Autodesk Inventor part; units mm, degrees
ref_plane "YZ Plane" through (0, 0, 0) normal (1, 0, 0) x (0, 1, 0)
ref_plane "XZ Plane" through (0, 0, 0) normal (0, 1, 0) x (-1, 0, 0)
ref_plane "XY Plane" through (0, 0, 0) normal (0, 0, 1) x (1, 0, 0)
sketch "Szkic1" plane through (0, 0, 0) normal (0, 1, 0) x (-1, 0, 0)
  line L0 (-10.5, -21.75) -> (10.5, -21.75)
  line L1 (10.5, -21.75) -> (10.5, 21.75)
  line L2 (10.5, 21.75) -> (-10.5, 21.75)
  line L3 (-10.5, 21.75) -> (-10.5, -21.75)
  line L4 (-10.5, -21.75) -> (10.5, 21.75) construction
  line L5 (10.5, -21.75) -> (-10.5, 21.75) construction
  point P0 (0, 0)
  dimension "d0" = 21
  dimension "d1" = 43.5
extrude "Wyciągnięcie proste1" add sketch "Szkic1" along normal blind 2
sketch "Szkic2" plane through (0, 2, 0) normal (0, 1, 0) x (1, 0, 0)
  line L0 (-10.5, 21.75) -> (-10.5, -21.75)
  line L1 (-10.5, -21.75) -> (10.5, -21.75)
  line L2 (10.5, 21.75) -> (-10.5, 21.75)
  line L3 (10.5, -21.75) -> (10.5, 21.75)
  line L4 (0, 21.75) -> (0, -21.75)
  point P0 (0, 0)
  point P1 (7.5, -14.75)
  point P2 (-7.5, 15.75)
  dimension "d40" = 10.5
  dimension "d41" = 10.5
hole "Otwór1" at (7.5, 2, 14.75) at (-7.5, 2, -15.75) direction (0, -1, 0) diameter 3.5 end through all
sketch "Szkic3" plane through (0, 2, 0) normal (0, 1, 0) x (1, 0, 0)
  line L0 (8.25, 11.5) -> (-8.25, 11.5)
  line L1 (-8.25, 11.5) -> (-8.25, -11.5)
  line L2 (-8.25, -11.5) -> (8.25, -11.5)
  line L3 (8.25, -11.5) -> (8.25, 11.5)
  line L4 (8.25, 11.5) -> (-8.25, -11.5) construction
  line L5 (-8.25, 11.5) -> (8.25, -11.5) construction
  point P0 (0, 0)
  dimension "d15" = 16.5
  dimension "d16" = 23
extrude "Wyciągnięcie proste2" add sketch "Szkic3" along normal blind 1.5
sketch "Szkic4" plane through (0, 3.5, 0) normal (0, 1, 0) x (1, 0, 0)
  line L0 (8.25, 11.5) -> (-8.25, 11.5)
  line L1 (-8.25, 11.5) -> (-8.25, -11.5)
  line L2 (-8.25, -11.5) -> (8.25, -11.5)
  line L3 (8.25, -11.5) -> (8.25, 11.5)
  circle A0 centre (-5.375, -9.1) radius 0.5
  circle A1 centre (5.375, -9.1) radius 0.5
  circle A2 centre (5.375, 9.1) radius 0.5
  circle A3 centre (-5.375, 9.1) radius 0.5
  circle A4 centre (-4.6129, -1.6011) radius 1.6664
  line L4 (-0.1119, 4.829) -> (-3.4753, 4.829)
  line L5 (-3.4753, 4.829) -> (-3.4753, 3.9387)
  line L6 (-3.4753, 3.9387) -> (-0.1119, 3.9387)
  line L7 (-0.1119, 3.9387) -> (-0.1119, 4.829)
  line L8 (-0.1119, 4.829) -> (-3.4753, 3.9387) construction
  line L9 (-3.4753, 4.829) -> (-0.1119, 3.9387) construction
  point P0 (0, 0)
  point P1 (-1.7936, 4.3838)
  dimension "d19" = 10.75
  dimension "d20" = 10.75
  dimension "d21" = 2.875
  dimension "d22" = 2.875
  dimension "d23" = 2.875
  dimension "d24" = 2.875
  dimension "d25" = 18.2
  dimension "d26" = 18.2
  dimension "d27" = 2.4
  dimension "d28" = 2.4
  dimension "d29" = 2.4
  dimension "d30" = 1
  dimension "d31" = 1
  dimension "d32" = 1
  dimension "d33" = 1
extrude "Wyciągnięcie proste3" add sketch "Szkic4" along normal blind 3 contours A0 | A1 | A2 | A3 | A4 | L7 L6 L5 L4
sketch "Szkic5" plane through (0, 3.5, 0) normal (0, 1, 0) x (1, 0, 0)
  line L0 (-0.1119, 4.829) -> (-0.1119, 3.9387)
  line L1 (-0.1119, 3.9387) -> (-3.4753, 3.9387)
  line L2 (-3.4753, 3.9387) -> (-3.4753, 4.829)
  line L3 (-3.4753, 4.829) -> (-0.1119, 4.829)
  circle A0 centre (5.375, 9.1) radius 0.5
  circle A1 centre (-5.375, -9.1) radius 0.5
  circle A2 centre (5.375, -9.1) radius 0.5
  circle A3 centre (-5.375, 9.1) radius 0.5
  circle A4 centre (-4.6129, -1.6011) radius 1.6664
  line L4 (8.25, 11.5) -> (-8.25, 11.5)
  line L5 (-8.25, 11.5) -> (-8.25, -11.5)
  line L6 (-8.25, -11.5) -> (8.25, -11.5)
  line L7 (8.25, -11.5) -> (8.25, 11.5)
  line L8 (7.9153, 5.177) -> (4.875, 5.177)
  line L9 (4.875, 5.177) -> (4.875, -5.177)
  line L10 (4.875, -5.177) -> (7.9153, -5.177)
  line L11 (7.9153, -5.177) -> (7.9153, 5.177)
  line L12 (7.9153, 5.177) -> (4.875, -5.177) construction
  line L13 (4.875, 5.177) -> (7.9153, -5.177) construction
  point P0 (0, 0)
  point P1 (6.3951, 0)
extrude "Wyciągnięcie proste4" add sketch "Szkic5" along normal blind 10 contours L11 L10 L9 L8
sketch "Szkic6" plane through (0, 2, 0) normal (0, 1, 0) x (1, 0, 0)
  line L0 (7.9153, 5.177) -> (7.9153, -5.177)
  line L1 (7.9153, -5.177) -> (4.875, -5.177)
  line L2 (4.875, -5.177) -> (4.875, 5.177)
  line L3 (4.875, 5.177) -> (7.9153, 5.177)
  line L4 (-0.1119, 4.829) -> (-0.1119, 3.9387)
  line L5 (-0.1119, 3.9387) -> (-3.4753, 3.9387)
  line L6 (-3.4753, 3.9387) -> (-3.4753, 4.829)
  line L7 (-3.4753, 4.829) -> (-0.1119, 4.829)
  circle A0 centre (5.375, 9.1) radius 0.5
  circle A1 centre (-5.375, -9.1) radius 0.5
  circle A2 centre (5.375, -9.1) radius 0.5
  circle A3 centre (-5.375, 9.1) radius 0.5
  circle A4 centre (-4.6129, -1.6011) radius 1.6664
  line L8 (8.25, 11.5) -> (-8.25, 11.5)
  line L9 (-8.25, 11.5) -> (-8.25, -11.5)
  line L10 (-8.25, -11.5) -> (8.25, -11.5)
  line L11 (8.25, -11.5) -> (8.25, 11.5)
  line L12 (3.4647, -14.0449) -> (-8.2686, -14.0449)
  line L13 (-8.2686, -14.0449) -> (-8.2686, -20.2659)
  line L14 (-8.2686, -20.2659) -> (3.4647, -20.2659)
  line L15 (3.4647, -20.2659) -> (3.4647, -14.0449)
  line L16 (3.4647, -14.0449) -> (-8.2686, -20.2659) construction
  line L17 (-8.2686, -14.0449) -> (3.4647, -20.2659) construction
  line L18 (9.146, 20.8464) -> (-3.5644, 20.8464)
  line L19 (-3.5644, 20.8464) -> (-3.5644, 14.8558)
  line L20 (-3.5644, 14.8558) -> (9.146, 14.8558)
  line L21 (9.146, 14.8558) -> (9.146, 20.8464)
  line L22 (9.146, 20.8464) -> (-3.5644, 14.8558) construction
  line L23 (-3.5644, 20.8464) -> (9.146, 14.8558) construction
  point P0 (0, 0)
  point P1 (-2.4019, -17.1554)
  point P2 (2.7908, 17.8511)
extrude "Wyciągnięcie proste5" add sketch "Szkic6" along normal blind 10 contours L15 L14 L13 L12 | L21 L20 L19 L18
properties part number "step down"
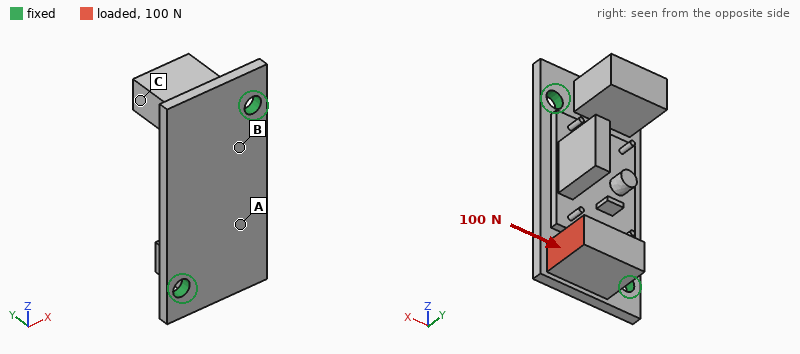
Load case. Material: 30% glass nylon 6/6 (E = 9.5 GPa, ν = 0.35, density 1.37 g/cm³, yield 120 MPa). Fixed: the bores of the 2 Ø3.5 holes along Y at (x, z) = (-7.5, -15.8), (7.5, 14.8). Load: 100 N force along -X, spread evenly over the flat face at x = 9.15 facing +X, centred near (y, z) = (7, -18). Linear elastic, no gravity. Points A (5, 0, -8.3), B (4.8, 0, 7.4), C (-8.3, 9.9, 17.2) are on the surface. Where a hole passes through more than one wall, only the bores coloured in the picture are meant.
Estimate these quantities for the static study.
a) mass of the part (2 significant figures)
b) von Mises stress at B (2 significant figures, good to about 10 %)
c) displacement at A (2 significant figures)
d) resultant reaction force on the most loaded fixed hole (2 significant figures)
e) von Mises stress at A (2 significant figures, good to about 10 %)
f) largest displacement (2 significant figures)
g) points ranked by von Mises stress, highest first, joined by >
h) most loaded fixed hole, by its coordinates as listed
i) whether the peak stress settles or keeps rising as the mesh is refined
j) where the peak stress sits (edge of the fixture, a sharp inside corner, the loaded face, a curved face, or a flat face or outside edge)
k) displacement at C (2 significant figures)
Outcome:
5.8 g
9.0 MPa
0.10 mm
95 N
12 MPa
0.31 mm
A > B > C
(-7.5, -15.8)
keeps rising
edge of the fixture
0.091 mm
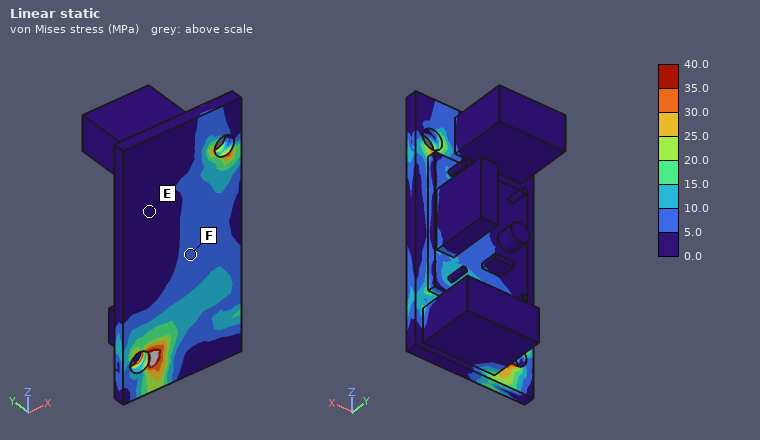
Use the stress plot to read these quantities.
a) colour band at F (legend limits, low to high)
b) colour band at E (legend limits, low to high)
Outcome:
5.0 to 10.0 MPa
0.0 to 5.0 MPa
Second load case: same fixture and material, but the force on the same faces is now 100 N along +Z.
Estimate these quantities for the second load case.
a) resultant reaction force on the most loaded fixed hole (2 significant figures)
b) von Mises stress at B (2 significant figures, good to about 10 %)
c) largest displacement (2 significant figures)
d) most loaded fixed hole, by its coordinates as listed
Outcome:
73 N
2.8 MPa
0.22 mm
(7.5, 14.8)
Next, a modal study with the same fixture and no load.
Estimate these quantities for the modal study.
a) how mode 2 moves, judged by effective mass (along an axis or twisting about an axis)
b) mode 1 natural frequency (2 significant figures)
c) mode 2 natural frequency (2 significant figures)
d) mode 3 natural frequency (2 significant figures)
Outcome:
along Y
1900 Hz
2800 Hz
4200 Hz
